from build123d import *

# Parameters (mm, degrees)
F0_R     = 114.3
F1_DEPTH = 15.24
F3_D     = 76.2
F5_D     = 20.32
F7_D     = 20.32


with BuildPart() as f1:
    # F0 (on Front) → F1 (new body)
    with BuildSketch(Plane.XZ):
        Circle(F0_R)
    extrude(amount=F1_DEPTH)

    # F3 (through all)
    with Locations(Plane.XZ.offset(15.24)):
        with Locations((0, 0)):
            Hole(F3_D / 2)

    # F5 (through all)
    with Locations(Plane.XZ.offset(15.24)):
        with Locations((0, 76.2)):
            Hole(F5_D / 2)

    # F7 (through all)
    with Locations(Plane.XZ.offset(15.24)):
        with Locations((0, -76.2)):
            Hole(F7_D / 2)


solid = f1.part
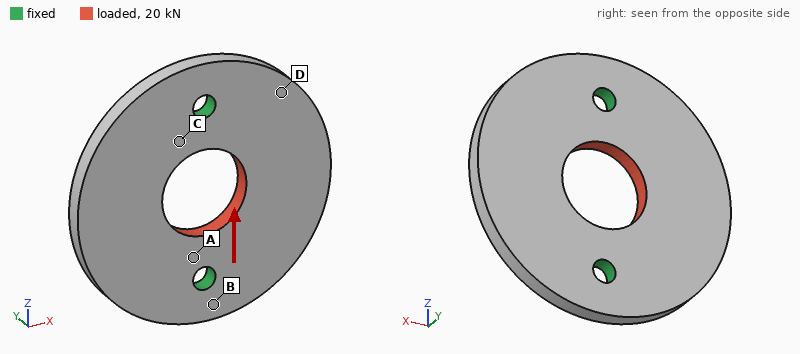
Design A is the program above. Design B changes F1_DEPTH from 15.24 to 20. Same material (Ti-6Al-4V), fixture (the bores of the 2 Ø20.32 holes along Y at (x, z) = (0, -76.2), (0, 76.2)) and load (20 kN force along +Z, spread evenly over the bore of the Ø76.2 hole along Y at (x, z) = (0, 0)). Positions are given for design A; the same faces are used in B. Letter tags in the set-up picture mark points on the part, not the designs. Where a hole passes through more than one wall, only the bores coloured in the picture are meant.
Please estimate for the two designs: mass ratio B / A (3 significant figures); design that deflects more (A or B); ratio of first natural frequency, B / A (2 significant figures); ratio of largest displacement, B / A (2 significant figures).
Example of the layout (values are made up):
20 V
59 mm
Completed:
1.31
A
1.3
0.76
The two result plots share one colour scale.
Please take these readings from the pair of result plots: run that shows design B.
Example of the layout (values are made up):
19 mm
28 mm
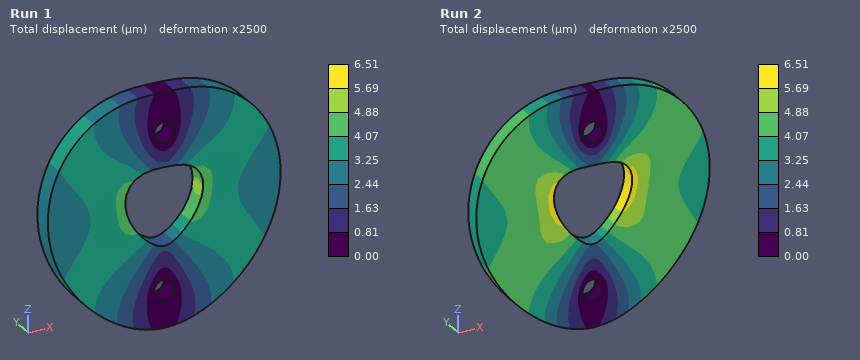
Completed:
Run 1
